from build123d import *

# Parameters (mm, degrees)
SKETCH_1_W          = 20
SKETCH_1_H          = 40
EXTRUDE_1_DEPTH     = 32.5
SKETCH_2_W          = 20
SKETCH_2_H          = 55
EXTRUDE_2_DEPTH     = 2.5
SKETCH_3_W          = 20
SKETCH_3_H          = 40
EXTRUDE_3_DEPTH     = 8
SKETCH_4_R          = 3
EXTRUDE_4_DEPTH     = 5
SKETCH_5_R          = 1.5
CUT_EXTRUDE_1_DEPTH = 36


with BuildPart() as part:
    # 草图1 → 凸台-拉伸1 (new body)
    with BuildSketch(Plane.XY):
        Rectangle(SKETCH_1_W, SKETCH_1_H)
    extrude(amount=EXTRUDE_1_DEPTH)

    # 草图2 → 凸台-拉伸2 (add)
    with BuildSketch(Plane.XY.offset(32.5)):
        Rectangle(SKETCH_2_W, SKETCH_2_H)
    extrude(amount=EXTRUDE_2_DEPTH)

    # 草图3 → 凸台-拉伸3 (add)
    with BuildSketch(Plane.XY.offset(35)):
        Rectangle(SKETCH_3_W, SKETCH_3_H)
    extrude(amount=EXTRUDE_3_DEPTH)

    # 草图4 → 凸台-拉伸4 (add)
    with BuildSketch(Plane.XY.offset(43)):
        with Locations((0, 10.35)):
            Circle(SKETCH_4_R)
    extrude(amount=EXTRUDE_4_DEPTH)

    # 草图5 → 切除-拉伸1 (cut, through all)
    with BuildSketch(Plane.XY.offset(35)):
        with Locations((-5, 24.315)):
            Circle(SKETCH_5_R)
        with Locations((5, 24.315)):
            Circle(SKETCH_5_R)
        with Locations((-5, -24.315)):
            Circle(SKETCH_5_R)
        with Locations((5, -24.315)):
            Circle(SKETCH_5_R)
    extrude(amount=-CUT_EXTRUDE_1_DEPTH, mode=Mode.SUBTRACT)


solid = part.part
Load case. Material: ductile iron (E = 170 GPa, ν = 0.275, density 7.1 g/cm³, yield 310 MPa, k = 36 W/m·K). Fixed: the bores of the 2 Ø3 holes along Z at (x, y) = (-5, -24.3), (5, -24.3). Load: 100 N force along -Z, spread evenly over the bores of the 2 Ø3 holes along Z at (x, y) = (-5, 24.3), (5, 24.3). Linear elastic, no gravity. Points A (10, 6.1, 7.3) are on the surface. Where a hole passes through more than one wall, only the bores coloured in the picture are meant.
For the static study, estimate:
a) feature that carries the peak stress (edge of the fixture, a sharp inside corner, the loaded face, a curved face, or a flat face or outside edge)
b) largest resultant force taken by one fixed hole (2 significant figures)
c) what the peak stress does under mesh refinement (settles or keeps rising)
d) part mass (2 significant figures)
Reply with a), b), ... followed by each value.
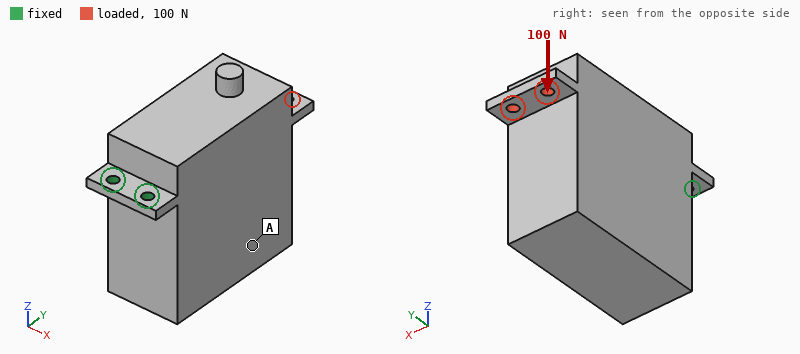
a) edge of the fixture
b) 50 N
c) keeps rising
d) 250 g
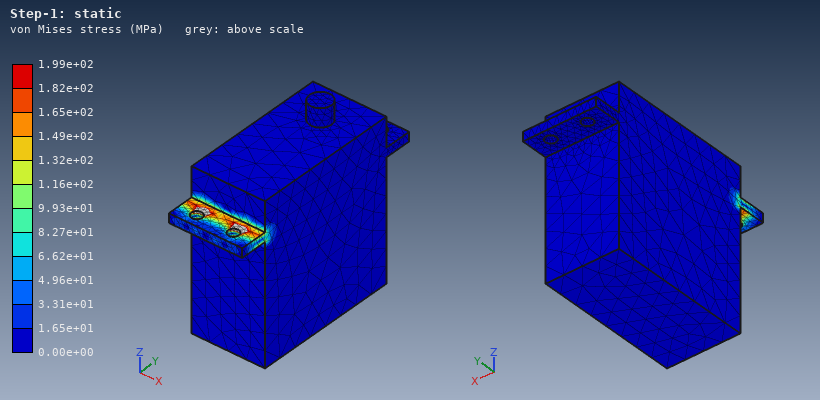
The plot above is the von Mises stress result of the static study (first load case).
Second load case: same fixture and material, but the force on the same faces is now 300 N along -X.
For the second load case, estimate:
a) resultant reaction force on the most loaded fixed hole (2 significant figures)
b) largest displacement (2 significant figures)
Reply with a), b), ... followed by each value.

a) 1.2 kN
b) 27 µm
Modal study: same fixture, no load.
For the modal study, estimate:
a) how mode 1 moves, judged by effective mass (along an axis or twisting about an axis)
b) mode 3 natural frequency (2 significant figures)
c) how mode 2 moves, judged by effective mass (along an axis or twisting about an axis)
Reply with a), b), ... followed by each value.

a) along Z
b) 2800 Hz
c) along X
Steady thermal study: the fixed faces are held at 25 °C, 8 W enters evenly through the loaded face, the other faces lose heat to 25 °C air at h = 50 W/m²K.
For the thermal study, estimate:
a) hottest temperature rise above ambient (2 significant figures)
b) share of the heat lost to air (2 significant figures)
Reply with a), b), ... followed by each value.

a) 52 K
b) 63 %
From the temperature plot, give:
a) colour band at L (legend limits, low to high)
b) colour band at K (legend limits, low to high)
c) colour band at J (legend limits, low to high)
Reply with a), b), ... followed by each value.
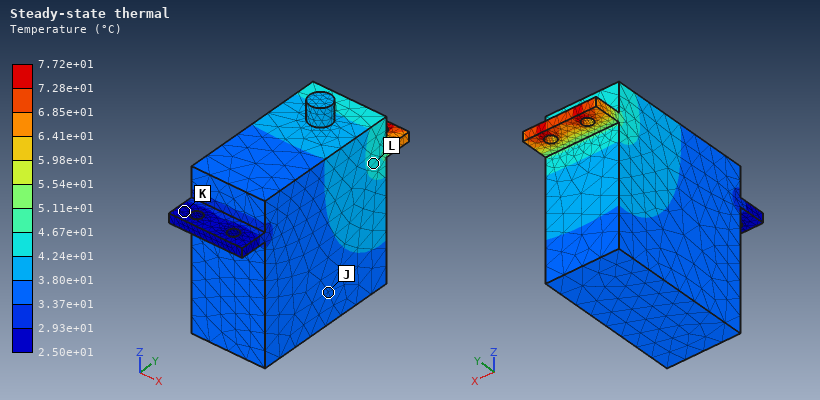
a) 4.24e+01 to 4.67e+01 °C
b) 2.50e+01 to 2.93e+01 °C
c) 3.37e+01 to 3.80e+01 °C
